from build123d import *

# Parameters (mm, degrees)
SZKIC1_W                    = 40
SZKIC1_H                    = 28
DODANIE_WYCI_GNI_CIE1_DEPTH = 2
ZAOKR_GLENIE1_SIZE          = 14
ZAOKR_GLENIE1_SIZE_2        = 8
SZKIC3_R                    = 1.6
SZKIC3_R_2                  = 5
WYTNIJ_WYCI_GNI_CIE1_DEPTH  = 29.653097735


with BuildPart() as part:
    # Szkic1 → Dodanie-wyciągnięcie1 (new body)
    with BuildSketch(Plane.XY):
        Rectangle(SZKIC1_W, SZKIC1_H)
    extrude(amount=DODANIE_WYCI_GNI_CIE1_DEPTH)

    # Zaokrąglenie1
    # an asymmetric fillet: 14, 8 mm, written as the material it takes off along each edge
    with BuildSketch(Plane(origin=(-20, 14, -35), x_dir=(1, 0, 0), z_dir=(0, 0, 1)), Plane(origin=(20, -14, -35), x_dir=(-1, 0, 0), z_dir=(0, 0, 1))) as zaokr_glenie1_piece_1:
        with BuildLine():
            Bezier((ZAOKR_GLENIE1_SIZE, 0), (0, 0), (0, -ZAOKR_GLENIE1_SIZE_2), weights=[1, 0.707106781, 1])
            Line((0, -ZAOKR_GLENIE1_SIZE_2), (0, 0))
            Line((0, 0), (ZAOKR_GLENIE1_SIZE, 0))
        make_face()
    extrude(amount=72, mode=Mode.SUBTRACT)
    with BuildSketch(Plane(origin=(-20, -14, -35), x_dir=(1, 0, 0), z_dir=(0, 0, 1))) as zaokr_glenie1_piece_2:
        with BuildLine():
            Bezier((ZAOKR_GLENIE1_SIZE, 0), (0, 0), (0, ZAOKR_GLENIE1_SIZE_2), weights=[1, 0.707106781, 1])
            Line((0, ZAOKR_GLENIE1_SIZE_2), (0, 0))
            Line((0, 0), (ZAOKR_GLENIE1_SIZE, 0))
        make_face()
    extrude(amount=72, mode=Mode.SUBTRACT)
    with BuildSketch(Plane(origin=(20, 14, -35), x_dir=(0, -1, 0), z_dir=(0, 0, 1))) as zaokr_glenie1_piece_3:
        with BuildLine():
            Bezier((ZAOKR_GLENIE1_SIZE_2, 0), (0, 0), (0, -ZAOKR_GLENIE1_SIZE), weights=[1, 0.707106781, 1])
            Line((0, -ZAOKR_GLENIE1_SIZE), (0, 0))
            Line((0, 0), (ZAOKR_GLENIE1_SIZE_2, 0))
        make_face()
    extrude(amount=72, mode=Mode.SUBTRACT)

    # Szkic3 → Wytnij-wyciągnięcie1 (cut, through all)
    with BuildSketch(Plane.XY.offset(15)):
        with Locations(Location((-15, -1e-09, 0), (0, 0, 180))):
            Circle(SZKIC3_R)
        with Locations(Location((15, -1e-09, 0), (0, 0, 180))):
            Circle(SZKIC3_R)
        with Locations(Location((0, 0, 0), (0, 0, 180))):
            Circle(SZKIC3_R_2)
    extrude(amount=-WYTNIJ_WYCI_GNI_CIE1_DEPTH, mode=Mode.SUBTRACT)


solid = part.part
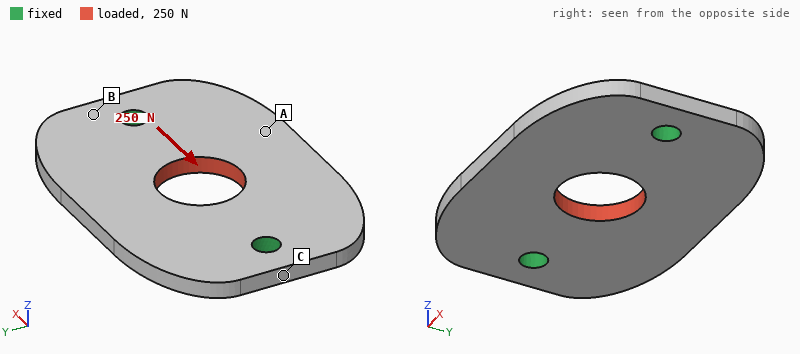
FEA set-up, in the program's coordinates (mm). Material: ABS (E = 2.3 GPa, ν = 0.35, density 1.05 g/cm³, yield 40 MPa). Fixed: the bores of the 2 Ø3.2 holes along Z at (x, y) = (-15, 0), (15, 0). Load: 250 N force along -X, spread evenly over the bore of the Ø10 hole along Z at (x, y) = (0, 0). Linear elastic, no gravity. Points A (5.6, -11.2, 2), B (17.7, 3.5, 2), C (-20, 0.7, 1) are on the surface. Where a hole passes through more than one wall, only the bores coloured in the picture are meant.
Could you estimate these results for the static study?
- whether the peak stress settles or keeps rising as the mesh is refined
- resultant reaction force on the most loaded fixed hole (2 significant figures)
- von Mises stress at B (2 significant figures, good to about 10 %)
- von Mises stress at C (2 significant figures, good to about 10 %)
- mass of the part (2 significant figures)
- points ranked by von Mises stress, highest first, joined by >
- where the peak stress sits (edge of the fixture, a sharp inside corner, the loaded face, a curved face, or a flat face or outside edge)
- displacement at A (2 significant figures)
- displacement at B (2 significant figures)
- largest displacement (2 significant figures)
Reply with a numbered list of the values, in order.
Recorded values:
1. keeps rising
2. 130 N
3. 2.5 MPa
4. 4.6 MPa
5. 2.0 g
6. C > B > A
7. edge of the fixture
8. 22 µm
9. 7.3 µm
10. 34 µm
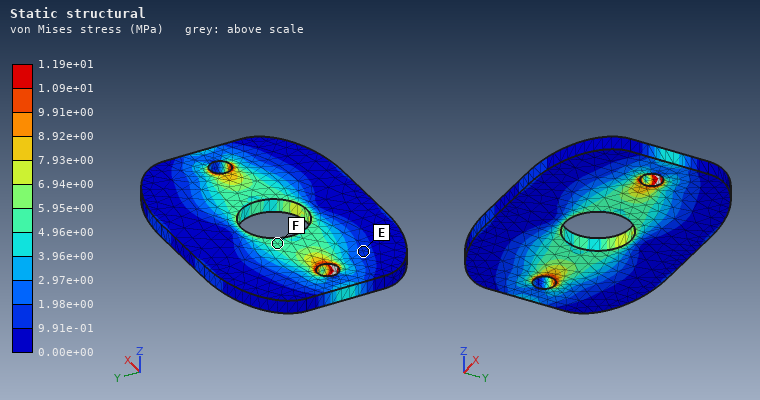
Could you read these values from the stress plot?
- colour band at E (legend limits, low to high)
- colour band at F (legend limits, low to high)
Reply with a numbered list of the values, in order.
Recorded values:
1. 9.91e-01 to 1.98e+00 MPa
2. 4.96e+00 to 5.95e+00 MPa
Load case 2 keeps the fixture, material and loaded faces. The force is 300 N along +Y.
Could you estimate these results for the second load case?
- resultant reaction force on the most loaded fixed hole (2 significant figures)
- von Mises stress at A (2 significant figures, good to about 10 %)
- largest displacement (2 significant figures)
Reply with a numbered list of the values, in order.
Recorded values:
1. 150 N
2. 5.0 MPa
3. 71 µm
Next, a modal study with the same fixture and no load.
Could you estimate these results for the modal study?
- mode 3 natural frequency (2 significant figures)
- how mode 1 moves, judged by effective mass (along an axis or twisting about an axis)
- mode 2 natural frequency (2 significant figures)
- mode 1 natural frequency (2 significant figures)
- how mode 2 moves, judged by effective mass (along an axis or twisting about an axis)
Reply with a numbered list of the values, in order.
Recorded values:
1. 4000 Hz
2. twisting about X
3. 2200 Hz
4. 1900 Hz
5. along Z
